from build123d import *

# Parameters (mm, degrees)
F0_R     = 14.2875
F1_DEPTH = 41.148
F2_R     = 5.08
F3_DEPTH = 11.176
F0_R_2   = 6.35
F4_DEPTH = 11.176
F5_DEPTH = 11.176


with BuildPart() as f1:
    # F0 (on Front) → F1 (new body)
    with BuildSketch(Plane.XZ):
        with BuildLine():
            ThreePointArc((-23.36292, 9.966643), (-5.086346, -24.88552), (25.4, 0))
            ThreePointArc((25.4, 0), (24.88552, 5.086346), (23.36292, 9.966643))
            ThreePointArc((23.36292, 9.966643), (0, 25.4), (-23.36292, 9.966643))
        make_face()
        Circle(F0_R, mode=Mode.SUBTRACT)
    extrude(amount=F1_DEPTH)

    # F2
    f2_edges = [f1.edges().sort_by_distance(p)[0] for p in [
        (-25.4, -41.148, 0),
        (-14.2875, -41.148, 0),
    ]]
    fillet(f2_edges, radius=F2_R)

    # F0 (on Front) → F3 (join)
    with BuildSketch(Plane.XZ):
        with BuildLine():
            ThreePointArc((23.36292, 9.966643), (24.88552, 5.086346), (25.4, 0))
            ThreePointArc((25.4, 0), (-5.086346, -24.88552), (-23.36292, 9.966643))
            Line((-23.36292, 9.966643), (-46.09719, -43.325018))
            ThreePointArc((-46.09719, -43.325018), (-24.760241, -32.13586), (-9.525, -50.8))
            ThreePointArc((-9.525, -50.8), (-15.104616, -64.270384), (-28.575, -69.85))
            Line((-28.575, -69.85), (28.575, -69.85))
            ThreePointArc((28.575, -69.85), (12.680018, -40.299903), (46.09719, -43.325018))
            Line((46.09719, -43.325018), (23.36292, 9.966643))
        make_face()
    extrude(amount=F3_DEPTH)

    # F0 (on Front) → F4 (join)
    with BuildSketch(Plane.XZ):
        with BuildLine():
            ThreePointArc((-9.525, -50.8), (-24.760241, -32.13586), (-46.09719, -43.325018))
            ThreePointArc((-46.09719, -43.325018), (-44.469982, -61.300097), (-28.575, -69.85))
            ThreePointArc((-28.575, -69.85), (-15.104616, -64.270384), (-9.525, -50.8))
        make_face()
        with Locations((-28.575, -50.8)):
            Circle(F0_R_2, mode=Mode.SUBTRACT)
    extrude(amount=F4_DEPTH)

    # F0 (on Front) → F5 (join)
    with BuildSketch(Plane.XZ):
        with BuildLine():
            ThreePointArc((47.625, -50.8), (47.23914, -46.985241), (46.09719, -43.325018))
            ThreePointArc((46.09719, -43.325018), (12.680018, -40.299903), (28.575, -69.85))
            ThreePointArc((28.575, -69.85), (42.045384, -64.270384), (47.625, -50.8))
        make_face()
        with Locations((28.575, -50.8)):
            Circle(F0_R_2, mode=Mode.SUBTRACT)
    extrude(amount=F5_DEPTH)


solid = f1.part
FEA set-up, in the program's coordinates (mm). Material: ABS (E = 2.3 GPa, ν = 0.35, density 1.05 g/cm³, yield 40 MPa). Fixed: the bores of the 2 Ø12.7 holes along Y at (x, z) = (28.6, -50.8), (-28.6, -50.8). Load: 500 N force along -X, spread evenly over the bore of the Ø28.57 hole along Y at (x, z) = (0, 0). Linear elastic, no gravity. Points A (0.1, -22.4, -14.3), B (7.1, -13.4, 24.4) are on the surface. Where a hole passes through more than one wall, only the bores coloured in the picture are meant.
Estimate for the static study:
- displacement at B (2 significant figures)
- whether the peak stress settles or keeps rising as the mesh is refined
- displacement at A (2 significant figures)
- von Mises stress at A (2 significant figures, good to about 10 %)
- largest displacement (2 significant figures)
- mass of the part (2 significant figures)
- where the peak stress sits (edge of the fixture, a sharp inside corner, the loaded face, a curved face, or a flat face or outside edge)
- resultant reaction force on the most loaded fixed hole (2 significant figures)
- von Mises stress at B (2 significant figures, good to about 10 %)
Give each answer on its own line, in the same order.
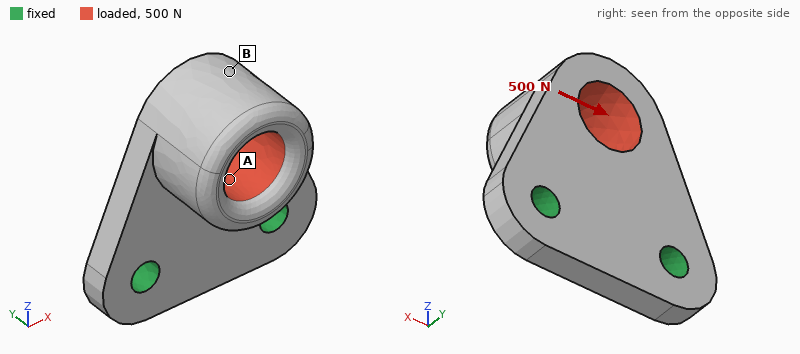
0.100 mm
keeps rising
0.076 mm
1.2 MPa
0.17 mm
110 g
edge of the fixture
470 N
0.41 MPa
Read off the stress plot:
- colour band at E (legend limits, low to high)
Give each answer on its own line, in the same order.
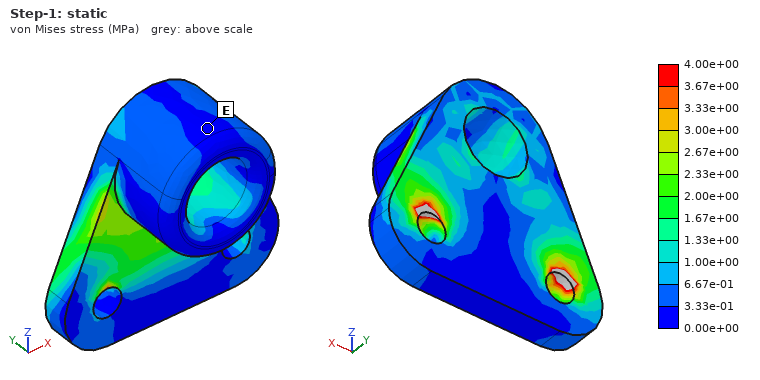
0.00e+00 to 3.33e-01 MPa
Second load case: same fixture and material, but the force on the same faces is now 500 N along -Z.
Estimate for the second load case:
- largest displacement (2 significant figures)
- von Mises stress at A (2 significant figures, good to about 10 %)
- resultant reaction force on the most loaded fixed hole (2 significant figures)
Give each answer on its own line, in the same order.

0.64 mm
0.73 MPa
260 N
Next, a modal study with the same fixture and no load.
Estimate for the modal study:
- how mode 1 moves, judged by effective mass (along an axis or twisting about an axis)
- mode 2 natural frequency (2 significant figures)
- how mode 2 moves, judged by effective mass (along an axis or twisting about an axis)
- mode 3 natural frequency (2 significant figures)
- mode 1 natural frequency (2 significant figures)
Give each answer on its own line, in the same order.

along Y
1100 Hz
along X
1900 Hz
400 Hz
